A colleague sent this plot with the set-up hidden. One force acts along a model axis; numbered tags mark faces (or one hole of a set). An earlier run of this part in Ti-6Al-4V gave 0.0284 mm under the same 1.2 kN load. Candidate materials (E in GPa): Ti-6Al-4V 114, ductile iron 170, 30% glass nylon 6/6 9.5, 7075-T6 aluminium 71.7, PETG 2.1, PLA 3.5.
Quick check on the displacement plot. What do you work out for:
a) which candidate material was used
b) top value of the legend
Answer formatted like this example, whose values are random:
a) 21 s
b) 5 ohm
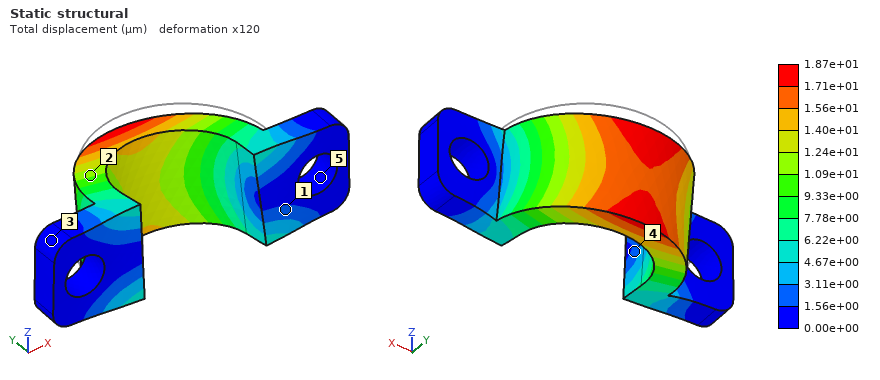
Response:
a) ductile iron
b) 1.87e+01 µm
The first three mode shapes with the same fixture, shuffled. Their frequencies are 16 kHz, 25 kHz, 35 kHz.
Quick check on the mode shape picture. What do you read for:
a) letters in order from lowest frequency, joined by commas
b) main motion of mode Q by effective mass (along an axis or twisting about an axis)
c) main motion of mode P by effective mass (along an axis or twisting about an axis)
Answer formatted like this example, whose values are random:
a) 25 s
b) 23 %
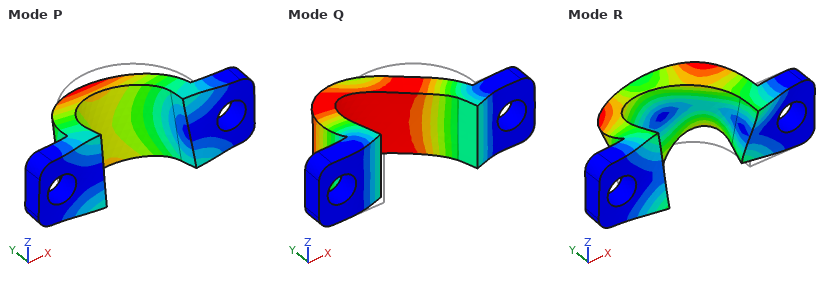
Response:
a) P, Q, R
b) along X
c) along Z
